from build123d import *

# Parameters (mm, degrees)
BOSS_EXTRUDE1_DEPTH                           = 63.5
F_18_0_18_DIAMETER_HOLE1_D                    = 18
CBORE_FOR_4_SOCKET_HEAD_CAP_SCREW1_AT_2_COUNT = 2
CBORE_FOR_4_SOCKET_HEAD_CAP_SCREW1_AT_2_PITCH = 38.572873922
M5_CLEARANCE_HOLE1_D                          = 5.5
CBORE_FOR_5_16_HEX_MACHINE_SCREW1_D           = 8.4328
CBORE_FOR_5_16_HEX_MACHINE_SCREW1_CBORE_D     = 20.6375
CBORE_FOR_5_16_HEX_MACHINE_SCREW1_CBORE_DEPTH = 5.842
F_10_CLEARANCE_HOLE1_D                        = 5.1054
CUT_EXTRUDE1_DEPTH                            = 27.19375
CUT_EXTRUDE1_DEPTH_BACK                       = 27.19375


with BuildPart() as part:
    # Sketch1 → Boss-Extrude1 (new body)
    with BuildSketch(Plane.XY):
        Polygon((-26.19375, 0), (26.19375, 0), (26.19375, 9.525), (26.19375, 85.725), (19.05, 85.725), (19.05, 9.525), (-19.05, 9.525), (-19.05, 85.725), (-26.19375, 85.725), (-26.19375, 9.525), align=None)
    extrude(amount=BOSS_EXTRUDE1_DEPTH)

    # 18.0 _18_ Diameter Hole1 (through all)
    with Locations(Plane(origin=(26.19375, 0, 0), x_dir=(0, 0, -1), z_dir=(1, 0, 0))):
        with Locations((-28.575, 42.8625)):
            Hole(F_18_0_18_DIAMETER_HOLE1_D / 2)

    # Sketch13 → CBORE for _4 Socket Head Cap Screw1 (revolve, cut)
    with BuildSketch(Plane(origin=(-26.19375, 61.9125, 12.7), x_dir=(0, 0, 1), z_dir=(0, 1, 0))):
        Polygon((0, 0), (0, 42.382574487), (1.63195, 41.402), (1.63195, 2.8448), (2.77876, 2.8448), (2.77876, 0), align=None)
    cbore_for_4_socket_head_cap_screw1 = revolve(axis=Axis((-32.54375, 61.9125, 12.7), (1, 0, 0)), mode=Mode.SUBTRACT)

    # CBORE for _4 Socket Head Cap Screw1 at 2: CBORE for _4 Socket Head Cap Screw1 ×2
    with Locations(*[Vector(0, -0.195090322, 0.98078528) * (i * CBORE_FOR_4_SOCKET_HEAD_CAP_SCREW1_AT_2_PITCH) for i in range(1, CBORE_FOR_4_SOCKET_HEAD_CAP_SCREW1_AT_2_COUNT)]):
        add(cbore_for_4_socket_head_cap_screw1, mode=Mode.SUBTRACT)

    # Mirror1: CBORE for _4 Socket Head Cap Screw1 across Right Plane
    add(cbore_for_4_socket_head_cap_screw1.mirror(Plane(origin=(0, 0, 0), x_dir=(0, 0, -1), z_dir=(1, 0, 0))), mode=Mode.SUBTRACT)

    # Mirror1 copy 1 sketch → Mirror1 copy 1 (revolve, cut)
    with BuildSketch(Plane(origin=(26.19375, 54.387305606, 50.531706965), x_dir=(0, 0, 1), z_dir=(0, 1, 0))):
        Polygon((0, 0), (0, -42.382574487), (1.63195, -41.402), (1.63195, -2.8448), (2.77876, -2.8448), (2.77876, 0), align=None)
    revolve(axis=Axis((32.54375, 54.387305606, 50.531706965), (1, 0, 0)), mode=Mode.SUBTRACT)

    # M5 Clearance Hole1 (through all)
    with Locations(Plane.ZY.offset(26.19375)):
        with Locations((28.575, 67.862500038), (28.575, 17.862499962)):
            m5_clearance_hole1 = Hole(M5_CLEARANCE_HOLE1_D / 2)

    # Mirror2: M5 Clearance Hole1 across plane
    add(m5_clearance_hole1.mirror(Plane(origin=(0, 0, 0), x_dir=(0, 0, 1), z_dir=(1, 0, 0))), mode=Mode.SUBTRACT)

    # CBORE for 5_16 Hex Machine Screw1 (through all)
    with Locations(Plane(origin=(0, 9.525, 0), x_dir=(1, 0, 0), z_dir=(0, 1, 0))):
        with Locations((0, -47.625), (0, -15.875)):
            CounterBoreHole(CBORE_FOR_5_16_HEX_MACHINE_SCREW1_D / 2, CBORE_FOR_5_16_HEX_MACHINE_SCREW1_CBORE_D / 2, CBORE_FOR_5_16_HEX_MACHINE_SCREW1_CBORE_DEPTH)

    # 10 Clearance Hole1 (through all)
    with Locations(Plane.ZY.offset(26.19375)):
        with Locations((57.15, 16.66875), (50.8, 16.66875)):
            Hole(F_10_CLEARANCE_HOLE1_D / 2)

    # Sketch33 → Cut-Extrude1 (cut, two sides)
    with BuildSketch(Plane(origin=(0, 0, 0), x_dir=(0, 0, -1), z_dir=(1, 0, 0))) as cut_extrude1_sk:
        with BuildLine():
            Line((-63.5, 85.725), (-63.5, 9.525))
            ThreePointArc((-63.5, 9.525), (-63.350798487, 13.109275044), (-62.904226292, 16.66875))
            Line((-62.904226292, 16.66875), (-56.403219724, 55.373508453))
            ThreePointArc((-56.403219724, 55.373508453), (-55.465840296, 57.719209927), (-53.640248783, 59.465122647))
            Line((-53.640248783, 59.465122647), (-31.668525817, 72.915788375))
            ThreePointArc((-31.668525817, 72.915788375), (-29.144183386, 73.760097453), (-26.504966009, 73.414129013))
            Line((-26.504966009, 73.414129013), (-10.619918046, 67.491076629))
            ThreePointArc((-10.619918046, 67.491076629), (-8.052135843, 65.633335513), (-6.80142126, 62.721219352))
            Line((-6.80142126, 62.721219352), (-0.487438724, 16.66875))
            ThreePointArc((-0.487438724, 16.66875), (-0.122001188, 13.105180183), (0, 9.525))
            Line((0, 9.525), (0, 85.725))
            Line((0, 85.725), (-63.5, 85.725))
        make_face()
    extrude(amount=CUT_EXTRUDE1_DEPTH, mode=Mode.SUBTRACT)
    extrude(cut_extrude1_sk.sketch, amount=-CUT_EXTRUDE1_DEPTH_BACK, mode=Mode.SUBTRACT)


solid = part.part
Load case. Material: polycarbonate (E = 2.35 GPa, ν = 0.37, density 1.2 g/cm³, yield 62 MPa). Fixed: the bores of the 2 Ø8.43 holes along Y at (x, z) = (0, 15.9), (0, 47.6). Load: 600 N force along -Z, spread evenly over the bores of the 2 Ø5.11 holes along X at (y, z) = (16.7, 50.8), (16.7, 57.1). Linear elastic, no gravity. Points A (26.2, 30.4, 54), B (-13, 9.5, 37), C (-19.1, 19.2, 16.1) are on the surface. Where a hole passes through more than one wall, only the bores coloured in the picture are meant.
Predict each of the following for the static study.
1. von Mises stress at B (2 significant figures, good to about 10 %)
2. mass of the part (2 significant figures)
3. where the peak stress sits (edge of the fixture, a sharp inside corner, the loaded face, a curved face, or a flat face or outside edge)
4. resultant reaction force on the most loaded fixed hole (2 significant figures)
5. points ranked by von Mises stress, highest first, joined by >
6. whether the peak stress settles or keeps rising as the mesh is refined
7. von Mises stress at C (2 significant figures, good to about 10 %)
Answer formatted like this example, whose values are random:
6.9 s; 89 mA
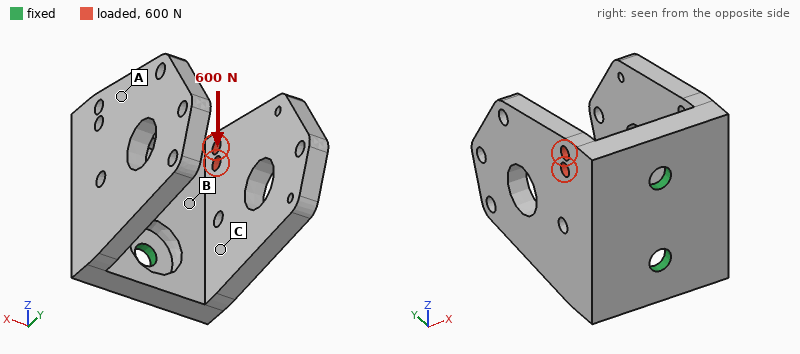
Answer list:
6.1 MPa; 82 g; edge of the fixture; 540 N; B > C > A; keeps rising; 2.8 MPa
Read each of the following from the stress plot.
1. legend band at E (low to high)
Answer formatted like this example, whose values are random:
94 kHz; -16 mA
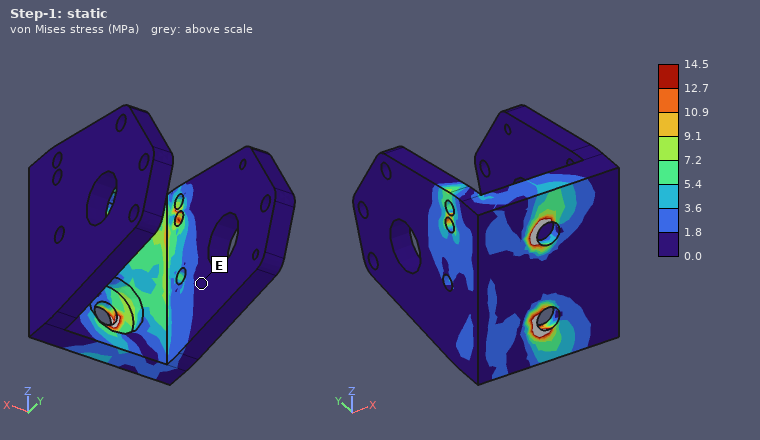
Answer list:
0.0 to 1.8 MPa
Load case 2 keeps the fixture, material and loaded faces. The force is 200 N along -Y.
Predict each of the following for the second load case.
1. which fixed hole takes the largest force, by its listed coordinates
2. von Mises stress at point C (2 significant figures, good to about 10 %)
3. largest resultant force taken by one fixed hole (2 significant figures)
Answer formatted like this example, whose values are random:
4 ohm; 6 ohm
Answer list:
(0, 47.6); 1.3 MPa; 220 N
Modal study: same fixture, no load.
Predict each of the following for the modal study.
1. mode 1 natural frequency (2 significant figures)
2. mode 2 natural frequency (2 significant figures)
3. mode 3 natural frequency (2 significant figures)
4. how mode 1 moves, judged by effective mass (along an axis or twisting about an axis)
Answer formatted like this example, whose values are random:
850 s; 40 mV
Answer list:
250 Hz; 350 Hz; 640 Hz; along X
